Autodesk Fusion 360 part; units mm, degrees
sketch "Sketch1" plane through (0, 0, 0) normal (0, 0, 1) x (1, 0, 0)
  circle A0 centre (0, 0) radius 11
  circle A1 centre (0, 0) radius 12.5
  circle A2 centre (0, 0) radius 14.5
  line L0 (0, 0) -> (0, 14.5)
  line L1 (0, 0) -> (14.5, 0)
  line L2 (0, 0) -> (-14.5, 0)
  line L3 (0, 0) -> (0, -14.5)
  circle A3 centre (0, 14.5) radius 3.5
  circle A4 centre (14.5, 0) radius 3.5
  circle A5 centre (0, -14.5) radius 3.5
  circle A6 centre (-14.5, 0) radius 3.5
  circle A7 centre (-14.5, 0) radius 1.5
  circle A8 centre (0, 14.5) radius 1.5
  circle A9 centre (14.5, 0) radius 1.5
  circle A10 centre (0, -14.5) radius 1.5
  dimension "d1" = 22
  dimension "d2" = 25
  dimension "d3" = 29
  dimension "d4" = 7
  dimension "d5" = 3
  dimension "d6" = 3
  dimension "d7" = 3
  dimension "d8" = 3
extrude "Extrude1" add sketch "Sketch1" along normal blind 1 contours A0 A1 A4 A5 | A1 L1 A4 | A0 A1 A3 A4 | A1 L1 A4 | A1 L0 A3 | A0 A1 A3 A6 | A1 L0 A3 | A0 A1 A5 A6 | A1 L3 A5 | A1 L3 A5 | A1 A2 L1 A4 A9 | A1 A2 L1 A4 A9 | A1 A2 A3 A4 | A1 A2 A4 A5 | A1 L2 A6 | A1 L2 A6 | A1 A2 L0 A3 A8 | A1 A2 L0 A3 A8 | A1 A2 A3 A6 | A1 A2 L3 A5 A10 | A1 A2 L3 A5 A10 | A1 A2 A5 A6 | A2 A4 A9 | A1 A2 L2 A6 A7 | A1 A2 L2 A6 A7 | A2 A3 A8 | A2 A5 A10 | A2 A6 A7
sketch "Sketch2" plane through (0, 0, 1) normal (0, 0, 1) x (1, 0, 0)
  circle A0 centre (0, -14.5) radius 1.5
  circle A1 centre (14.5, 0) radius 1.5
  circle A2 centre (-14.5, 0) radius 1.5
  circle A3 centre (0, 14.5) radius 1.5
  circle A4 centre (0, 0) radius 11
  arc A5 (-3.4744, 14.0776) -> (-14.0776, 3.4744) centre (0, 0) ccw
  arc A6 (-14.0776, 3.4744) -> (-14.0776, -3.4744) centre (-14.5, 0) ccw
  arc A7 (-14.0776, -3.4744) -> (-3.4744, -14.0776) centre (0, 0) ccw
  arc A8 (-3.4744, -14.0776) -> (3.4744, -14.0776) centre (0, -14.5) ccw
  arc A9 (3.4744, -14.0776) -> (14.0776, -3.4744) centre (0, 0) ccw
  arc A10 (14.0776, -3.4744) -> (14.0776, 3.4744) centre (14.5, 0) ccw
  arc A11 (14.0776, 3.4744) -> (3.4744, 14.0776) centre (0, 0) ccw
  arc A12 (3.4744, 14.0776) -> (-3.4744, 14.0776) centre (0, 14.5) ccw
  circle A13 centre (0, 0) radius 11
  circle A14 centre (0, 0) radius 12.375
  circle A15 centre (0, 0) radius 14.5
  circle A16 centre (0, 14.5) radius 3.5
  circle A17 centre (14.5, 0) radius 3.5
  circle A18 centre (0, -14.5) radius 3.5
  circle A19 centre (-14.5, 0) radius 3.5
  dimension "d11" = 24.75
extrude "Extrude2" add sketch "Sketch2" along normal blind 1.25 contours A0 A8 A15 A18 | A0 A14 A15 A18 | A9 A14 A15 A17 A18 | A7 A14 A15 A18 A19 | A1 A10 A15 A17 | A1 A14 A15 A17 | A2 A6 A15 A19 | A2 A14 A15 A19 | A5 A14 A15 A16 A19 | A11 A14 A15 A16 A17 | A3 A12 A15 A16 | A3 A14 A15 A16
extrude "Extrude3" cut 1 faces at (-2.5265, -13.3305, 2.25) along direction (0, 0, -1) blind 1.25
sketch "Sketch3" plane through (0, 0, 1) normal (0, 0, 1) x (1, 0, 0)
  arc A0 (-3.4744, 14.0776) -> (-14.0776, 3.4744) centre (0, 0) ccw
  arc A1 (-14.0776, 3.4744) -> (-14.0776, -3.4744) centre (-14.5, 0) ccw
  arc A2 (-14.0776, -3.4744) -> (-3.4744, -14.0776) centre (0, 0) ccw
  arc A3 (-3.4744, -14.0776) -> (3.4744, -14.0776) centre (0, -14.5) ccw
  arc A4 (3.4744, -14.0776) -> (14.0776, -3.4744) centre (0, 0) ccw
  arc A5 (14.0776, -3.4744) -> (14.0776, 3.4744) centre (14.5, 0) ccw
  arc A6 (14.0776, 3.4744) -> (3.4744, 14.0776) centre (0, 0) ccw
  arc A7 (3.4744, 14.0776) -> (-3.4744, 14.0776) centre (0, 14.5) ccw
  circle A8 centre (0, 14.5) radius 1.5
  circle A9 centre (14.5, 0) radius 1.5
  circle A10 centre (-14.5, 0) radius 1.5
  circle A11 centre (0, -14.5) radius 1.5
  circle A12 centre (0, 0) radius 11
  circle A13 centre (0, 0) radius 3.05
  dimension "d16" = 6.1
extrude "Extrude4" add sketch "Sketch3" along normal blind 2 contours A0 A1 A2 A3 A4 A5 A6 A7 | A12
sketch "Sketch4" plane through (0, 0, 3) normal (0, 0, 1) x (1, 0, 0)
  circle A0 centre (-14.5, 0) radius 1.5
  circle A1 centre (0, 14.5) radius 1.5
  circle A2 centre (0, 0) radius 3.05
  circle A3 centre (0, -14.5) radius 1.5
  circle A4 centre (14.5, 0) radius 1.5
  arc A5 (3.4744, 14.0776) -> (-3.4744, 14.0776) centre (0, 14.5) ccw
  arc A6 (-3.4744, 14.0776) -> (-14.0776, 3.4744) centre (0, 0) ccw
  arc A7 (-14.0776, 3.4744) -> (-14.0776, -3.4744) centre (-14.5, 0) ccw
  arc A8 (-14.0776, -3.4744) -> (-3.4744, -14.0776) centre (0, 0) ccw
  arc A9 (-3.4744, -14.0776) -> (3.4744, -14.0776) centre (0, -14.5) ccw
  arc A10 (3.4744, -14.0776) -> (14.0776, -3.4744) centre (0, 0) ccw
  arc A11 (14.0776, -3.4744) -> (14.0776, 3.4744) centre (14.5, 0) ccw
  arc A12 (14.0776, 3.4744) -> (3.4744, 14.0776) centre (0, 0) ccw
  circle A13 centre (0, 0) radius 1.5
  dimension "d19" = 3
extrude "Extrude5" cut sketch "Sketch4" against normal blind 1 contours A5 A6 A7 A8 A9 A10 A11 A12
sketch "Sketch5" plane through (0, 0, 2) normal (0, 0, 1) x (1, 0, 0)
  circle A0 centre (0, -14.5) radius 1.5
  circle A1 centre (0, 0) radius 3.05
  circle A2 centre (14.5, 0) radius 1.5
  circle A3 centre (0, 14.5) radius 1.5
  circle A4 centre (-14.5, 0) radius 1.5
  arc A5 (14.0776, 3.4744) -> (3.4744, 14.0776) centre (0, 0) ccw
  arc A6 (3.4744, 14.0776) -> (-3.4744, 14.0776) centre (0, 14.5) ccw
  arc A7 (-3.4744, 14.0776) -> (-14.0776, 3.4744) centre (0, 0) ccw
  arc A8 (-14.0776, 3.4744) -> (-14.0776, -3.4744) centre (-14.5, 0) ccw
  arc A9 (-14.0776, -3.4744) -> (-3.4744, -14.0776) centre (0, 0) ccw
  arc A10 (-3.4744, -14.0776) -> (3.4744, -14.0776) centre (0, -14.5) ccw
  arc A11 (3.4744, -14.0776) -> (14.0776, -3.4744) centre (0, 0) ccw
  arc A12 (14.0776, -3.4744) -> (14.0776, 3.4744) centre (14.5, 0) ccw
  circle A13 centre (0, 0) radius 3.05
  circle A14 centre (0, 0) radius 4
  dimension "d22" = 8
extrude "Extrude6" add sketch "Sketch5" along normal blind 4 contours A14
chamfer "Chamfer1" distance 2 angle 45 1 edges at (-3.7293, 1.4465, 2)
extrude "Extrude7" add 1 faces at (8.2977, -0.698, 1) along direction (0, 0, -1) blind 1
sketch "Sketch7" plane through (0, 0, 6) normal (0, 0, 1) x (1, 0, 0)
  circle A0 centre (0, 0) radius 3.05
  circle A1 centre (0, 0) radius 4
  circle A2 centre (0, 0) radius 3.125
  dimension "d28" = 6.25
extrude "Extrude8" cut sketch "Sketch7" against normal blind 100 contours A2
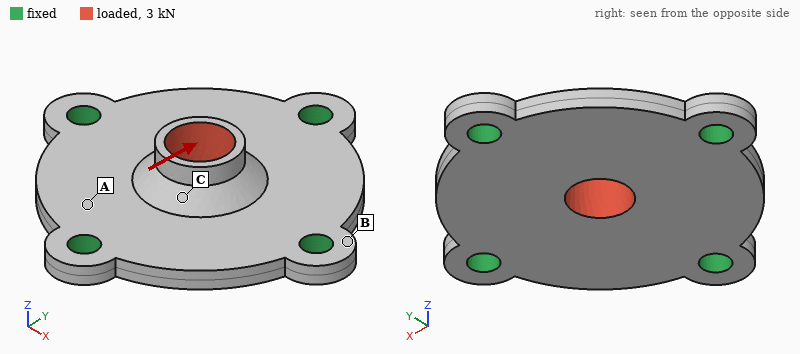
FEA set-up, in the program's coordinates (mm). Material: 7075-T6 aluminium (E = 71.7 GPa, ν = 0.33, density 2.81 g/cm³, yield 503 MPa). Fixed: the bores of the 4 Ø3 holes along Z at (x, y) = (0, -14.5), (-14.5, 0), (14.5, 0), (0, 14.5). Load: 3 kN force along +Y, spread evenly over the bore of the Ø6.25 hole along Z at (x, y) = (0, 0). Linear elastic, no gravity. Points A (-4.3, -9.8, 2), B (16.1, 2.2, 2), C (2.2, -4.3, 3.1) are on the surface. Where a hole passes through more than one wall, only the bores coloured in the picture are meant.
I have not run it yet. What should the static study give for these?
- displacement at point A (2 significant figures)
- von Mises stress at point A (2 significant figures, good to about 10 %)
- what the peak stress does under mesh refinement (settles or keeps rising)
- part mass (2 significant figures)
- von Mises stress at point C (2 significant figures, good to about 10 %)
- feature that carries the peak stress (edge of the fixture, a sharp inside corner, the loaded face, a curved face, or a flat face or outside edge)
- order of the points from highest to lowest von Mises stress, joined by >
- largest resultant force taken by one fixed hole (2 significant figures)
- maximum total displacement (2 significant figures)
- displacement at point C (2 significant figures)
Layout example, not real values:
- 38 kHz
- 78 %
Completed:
- 11 µm
- 61 MPa
- keeps rising
- 4.2 g
- 110 MPa
- edge of the fixture
- C > A > B
- 1.1 kN
- 41 µm
- 23 µm
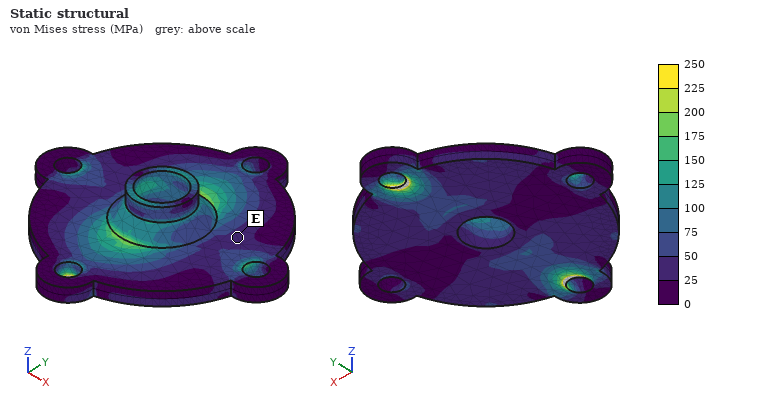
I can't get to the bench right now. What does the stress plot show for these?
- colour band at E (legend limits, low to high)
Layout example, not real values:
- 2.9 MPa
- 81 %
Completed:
- 25 to 50 MPa
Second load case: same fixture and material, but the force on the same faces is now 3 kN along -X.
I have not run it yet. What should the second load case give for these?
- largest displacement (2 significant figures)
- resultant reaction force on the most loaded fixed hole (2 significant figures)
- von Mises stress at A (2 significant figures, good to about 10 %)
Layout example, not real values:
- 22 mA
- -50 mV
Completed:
- 41 µm
- 1.1 kN
- 25 MPa
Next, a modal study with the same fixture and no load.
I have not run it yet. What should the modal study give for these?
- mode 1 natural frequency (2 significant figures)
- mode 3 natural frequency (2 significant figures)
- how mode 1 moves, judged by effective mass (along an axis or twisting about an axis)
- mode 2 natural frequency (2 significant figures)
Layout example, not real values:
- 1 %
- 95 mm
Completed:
- 20 kHz
- 27 kHz
- along Z
- 27 kHz
